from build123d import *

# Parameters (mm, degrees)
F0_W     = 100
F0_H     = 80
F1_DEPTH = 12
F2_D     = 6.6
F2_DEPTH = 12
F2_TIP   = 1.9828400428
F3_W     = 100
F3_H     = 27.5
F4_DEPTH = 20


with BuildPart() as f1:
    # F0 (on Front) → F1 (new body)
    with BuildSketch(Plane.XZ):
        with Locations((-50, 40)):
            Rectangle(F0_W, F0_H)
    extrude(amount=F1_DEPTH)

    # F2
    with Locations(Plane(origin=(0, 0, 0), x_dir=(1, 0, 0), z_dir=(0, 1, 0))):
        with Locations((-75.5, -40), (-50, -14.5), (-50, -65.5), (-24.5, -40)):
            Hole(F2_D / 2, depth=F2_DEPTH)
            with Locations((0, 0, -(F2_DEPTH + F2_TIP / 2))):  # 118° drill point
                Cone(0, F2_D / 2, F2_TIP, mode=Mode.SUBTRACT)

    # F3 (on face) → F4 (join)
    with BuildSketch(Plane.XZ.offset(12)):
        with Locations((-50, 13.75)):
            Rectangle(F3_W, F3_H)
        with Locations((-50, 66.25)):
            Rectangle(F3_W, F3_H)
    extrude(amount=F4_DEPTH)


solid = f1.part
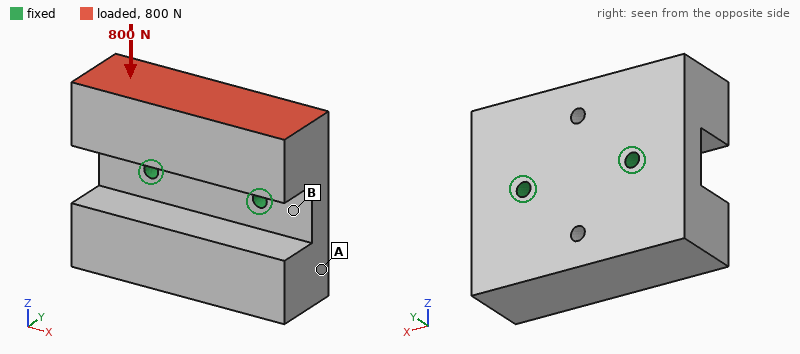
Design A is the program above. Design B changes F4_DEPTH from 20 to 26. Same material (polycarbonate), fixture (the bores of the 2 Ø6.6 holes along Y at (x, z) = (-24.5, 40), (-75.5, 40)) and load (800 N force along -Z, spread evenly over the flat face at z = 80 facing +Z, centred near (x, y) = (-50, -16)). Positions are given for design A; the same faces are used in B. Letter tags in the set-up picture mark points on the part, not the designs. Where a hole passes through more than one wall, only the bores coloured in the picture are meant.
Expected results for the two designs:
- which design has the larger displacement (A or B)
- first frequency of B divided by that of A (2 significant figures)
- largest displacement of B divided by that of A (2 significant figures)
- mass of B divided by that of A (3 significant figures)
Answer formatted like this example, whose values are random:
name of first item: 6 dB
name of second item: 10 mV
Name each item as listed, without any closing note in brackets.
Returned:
which design has the larger displacement: B
first frequency of B divided by that of A: 0.86
largest displacement of B divided by that of A: 1.4
mass of B divided by that of A: 1.16
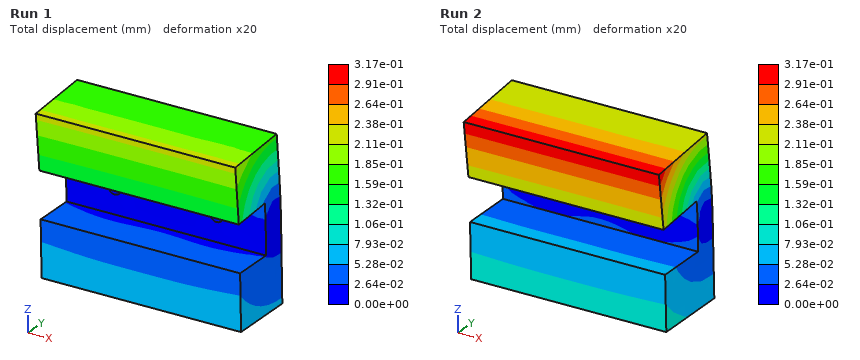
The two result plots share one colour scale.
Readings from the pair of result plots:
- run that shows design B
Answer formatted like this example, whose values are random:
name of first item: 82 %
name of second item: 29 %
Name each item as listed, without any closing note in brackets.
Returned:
run that shows design B: Run 2
